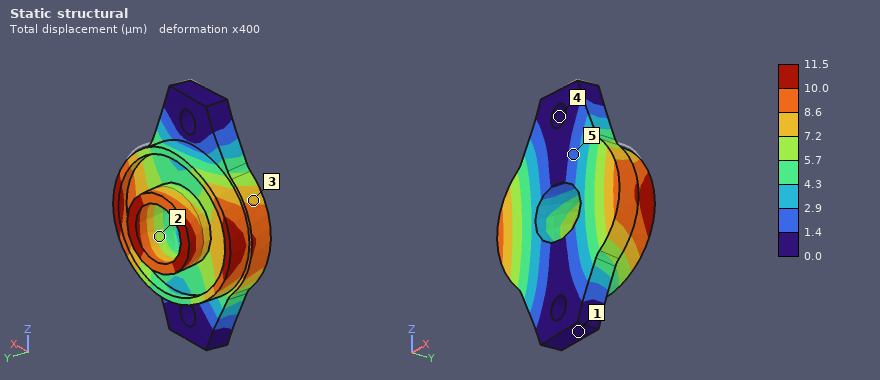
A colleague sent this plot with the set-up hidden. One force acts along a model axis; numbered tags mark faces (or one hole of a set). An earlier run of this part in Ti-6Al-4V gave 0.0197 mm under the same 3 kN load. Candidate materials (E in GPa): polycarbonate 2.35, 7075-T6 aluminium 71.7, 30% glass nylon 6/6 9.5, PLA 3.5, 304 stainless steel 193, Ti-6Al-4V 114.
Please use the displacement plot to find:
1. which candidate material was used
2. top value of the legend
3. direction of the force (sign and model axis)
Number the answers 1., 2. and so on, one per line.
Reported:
1. 304 stainless steel
2. 11.5 µm
3. -X
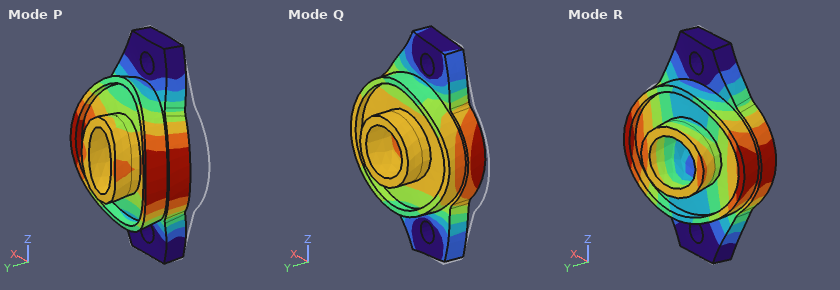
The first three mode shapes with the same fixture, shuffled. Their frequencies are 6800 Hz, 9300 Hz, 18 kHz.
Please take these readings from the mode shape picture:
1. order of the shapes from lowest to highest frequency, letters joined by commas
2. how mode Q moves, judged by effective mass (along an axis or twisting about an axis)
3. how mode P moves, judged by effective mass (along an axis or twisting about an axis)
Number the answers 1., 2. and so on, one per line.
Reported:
1. R, P, Q
2. along X
3. along Y
